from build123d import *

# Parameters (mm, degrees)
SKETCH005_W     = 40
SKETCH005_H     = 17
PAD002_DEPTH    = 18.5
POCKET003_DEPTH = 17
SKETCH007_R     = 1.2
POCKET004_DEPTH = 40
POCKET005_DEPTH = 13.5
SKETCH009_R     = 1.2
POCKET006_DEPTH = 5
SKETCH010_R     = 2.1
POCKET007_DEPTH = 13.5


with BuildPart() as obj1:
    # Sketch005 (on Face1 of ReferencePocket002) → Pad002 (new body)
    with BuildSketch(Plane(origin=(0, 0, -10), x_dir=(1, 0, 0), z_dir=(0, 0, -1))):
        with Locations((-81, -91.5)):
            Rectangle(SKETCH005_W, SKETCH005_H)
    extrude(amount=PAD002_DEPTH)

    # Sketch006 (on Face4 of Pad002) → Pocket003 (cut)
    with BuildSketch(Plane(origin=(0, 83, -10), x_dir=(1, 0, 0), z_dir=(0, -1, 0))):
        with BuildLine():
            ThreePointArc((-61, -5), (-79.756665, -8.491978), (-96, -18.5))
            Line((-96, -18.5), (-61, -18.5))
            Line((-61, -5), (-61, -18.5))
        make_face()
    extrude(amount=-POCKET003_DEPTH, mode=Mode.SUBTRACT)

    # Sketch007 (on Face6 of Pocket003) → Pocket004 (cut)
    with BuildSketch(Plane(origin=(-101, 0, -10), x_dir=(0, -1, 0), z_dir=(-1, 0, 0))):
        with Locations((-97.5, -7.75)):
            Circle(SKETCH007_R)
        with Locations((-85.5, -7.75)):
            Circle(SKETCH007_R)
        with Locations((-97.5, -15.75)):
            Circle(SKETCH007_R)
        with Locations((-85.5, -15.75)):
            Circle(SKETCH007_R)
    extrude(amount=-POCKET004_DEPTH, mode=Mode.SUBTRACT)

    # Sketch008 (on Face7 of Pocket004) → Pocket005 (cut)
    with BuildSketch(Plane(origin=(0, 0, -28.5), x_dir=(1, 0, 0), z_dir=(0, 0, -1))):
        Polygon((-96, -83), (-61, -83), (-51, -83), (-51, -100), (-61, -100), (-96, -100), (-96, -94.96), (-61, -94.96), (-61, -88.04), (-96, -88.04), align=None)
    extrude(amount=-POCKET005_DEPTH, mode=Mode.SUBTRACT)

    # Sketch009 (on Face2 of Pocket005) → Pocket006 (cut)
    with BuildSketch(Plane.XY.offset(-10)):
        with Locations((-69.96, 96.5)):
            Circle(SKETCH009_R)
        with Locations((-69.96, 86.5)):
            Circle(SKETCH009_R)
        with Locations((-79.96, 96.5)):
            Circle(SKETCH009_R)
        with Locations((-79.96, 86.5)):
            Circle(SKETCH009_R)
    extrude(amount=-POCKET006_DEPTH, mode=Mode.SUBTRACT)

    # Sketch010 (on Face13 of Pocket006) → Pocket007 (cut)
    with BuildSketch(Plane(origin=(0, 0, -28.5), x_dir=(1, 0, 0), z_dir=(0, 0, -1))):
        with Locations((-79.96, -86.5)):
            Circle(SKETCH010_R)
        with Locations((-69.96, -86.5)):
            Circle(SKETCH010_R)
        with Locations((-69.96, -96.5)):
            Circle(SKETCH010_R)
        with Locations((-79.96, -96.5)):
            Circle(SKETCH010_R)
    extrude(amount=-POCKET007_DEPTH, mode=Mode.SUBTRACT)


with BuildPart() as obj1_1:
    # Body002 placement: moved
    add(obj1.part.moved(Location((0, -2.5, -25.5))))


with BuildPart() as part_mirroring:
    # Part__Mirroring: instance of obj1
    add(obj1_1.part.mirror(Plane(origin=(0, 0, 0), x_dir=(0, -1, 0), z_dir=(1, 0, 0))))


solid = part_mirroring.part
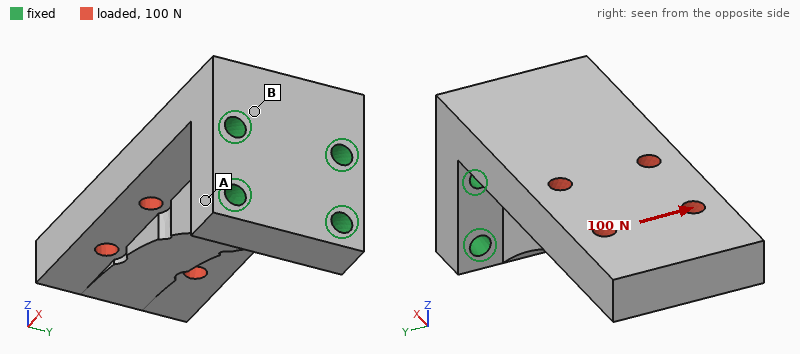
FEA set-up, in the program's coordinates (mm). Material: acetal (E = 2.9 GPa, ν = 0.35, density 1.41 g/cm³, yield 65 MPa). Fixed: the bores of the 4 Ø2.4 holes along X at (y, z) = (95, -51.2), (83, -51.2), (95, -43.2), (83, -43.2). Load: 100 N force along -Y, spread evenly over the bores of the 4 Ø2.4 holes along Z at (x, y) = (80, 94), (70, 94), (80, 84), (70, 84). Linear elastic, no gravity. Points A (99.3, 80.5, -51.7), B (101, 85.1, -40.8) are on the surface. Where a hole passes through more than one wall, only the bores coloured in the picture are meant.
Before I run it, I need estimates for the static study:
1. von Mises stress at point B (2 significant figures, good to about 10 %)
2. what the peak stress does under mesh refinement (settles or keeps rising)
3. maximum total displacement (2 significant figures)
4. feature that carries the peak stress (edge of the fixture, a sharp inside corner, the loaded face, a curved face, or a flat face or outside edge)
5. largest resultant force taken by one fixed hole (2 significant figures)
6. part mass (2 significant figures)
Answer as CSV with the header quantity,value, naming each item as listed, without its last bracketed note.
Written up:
quantity,value
von Mises stress at point B,4.6 MPa
what the peak stress does under mesh refinement,keeps rising
maximum total displacement,0.26 mm
feature that carries the peak stress,edge of the fixture
largest resultant force taken by one fixed hole,170 N
part mass,7.6 g
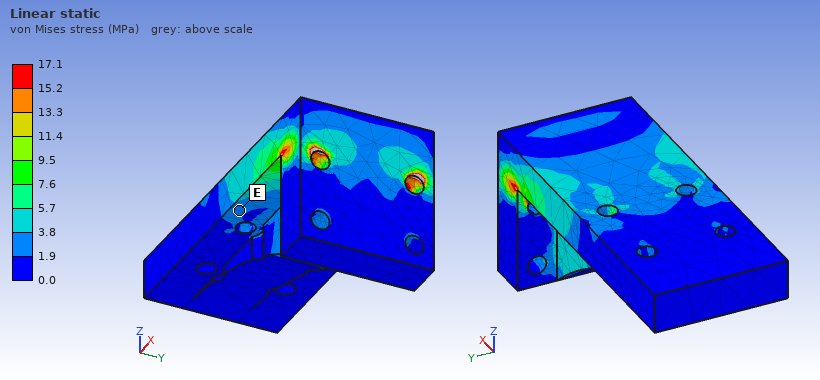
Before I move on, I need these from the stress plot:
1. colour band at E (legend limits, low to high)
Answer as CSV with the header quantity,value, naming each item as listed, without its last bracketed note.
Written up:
quantity,value
colour band at E,1.9 to 3.8 MPa
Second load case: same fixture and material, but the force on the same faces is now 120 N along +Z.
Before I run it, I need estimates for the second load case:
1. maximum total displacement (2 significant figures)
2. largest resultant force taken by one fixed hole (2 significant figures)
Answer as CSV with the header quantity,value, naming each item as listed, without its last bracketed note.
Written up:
quantity,value
maximum total displacement,0.38 mm
largest resultant force taken by one fixed hole,120 N
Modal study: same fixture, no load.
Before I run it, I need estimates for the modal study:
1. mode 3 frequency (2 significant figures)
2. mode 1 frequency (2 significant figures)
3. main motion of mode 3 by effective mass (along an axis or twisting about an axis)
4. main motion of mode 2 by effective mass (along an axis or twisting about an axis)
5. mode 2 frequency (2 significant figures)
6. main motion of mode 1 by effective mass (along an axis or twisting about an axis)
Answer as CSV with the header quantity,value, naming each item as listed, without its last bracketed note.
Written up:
quantity,value
mode 3 frequency,4500 Hz
mode 1 frequency,1800 Hz
main motion of mode 3 by effective mass,twisting about X
main motion of mode 2 by effective mass,along Y
mode 2 frequency,2000 Hz
main motion of mode 1 by effective mass,along Z
